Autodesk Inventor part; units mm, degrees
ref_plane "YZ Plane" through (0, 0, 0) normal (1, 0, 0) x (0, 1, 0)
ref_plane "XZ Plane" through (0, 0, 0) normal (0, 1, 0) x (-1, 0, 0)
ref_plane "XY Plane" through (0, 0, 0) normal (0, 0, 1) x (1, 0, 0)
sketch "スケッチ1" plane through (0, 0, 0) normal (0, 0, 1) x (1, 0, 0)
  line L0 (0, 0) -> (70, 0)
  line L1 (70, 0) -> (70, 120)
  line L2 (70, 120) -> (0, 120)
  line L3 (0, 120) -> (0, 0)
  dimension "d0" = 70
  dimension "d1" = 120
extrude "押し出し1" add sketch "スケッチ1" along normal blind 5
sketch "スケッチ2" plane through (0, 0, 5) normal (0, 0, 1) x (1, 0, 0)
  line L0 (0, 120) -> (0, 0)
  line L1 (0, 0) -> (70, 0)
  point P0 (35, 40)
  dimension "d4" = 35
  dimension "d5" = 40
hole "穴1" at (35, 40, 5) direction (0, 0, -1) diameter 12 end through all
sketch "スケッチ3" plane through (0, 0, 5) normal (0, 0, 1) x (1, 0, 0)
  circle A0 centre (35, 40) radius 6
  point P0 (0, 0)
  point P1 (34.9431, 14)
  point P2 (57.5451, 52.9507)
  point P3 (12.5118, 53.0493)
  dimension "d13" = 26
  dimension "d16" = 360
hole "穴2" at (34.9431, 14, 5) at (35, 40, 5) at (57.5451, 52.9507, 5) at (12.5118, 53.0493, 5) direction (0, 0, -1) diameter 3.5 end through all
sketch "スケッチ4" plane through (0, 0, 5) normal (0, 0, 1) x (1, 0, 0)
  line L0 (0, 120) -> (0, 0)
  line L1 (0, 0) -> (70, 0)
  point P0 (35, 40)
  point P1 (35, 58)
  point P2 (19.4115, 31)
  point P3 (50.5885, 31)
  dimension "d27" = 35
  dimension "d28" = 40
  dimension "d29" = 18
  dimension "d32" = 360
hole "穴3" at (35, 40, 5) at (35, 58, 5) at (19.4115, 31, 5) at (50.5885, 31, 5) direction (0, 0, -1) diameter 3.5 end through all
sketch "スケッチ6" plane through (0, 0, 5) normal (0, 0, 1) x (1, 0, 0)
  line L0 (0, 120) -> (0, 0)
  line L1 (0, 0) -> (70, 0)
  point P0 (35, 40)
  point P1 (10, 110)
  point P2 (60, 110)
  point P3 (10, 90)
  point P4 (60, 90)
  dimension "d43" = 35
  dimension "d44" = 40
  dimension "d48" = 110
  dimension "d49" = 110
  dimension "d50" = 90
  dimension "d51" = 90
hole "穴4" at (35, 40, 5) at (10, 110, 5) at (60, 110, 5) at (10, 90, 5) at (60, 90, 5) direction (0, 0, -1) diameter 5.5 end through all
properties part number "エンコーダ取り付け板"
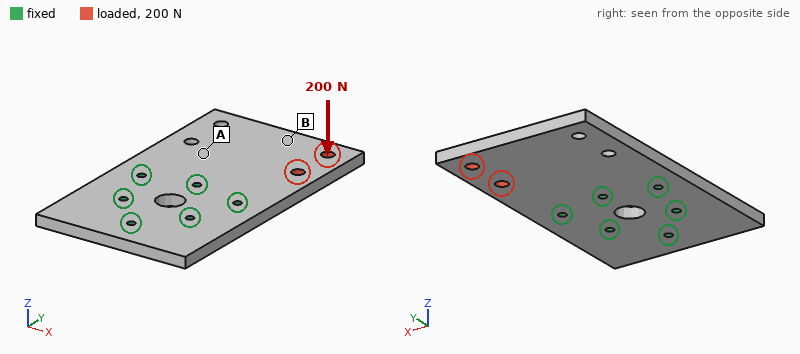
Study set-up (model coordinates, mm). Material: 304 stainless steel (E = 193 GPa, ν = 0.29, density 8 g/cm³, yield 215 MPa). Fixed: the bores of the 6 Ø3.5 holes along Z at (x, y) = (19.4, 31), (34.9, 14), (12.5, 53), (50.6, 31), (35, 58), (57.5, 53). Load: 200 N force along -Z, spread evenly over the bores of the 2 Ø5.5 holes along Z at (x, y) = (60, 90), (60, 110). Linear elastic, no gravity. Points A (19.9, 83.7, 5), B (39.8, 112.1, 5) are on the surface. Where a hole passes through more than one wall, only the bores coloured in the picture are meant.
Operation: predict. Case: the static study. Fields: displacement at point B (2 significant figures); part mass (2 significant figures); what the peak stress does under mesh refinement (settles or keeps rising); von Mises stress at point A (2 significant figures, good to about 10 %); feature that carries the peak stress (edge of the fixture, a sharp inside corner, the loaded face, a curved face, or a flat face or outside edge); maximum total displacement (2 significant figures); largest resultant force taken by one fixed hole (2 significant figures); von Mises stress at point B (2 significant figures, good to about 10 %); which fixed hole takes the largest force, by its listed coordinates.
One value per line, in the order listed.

0.064 mm
330 g
keeps rising
16 MPa
edge of the fixture
0.10 mm
230 N
7.8 MPa
(35, 58)
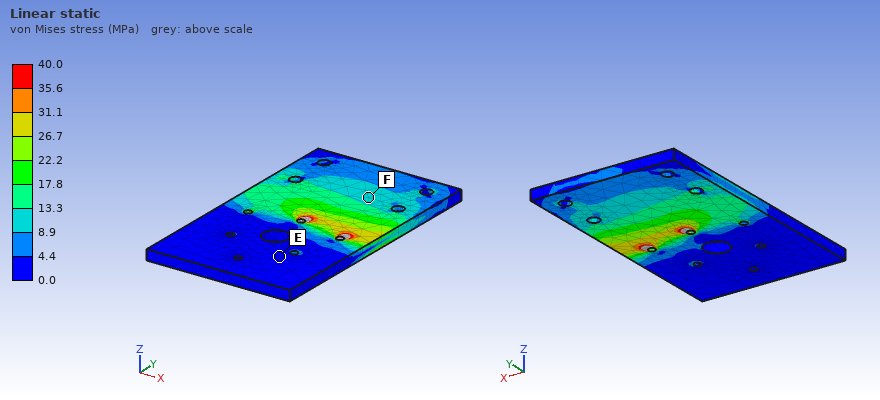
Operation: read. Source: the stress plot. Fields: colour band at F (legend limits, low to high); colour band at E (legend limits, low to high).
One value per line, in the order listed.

8.9 to 13.3 MPa
0.0 to 4.4 MPa
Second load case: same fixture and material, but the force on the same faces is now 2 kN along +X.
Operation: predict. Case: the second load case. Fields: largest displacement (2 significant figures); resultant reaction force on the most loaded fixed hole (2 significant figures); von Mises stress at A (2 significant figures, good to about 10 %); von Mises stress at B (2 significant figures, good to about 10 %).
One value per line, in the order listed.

12 µm
1.6 kN
10 MPa
6.9 MPa
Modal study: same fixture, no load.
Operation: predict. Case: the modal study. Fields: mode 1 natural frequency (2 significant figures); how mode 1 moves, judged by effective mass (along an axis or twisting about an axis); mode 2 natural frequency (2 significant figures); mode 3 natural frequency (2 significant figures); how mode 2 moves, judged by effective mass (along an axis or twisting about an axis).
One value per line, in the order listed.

950 Hz
along Z
2100 Hz
5200 Hz
twisting about Y
